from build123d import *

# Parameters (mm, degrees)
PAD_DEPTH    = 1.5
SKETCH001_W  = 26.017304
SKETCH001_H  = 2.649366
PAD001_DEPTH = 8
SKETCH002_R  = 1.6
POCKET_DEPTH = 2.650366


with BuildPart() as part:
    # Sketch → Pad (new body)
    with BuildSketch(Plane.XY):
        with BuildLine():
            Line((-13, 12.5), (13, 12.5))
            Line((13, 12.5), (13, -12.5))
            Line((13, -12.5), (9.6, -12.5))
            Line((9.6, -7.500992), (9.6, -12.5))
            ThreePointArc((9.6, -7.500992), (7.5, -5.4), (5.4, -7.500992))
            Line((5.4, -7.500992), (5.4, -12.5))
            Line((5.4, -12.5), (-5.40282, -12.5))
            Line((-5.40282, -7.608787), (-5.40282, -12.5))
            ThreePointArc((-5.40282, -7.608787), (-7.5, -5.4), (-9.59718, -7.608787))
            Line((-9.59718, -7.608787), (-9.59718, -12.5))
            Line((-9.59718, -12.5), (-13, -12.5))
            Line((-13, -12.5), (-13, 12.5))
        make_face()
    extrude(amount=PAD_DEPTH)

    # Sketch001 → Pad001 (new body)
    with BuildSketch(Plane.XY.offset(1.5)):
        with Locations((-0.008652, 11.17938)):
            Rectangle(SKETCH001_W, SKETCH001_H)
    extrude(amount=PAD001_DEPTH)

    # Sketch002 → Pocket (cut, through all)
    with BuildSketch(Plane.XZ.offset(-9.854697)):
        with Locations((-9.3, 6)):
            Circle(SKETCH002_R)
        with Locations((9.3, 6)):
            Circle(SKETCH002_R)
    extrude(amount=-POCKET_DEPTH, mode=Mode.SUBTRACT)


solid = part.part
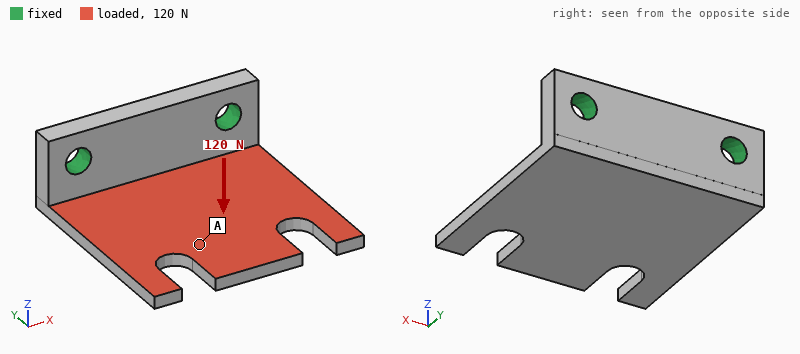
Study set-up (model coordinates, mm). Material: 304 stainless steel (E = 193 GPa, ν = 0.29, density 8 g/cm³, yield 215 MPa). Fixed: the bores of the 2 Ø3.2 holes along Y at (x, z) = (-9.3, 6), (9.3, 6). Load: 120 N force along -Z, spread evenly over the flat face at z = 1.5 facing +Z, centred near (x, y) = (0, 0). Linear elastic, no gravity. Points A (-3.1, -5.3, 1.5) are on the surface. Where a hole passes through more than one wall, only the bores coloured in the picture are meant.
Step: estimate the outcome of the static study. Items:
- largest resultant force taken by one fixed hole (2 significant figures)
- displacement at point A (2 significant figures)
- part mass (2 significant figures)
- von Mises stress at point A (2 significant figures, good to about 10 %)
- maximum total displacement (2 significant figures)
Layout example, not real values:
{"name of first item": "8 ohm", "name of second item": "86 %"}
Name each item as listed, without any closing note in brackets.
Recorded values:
{"largest resultant force taken by one fixed hole": "62 N", "displacement at point A": "0.081 mm", "part mass": "11 g", "von Mises stress at point A": "15 MPa", "maximum total displacement": "0.13 mm"}
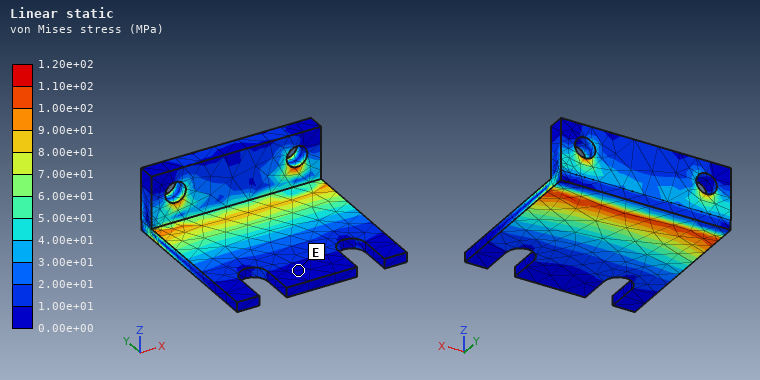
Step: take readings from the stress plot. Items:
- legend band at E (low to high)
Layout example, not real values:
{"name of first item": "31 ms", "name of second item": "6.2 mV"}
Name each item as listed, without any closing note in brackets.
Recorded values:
{"legend band at E": "0.00e+00 to 1.00e+01 MPa"}
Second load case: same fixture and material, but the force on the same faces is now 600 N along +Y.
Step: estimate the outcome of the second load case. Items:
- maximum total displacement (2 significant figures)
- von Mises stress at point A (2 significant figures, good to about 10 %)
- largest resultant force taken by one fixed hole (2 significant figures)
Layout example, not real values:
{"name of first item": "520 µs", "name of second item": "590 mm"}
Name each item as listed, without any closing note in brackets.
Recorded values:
{"maximum total displacement": "36 µm", "von Mises stress at point A": "19 MPa", "largest resultant force taken by one fixed hole": "300 N"}
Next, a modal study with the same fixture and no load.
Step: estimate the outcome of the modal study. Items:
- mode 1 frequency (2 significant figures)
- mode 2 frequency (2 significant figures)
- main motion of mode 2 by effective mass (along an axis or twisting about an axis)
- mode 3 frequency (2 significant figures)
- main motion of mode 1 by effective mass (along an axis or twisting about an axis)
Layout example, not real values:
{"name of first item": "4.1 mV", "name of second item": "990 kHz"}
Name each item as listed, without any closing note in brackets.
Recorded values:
{"mode 1 frequency": "2400 Hz", "mode 2 frequency": "4900 Hz", "main motion of mode 2 by effective mass": "twisting about Y", "mode 3 frequency": "9200 Hz", "main motion of mode 1 by effective mass": "along Z"}
